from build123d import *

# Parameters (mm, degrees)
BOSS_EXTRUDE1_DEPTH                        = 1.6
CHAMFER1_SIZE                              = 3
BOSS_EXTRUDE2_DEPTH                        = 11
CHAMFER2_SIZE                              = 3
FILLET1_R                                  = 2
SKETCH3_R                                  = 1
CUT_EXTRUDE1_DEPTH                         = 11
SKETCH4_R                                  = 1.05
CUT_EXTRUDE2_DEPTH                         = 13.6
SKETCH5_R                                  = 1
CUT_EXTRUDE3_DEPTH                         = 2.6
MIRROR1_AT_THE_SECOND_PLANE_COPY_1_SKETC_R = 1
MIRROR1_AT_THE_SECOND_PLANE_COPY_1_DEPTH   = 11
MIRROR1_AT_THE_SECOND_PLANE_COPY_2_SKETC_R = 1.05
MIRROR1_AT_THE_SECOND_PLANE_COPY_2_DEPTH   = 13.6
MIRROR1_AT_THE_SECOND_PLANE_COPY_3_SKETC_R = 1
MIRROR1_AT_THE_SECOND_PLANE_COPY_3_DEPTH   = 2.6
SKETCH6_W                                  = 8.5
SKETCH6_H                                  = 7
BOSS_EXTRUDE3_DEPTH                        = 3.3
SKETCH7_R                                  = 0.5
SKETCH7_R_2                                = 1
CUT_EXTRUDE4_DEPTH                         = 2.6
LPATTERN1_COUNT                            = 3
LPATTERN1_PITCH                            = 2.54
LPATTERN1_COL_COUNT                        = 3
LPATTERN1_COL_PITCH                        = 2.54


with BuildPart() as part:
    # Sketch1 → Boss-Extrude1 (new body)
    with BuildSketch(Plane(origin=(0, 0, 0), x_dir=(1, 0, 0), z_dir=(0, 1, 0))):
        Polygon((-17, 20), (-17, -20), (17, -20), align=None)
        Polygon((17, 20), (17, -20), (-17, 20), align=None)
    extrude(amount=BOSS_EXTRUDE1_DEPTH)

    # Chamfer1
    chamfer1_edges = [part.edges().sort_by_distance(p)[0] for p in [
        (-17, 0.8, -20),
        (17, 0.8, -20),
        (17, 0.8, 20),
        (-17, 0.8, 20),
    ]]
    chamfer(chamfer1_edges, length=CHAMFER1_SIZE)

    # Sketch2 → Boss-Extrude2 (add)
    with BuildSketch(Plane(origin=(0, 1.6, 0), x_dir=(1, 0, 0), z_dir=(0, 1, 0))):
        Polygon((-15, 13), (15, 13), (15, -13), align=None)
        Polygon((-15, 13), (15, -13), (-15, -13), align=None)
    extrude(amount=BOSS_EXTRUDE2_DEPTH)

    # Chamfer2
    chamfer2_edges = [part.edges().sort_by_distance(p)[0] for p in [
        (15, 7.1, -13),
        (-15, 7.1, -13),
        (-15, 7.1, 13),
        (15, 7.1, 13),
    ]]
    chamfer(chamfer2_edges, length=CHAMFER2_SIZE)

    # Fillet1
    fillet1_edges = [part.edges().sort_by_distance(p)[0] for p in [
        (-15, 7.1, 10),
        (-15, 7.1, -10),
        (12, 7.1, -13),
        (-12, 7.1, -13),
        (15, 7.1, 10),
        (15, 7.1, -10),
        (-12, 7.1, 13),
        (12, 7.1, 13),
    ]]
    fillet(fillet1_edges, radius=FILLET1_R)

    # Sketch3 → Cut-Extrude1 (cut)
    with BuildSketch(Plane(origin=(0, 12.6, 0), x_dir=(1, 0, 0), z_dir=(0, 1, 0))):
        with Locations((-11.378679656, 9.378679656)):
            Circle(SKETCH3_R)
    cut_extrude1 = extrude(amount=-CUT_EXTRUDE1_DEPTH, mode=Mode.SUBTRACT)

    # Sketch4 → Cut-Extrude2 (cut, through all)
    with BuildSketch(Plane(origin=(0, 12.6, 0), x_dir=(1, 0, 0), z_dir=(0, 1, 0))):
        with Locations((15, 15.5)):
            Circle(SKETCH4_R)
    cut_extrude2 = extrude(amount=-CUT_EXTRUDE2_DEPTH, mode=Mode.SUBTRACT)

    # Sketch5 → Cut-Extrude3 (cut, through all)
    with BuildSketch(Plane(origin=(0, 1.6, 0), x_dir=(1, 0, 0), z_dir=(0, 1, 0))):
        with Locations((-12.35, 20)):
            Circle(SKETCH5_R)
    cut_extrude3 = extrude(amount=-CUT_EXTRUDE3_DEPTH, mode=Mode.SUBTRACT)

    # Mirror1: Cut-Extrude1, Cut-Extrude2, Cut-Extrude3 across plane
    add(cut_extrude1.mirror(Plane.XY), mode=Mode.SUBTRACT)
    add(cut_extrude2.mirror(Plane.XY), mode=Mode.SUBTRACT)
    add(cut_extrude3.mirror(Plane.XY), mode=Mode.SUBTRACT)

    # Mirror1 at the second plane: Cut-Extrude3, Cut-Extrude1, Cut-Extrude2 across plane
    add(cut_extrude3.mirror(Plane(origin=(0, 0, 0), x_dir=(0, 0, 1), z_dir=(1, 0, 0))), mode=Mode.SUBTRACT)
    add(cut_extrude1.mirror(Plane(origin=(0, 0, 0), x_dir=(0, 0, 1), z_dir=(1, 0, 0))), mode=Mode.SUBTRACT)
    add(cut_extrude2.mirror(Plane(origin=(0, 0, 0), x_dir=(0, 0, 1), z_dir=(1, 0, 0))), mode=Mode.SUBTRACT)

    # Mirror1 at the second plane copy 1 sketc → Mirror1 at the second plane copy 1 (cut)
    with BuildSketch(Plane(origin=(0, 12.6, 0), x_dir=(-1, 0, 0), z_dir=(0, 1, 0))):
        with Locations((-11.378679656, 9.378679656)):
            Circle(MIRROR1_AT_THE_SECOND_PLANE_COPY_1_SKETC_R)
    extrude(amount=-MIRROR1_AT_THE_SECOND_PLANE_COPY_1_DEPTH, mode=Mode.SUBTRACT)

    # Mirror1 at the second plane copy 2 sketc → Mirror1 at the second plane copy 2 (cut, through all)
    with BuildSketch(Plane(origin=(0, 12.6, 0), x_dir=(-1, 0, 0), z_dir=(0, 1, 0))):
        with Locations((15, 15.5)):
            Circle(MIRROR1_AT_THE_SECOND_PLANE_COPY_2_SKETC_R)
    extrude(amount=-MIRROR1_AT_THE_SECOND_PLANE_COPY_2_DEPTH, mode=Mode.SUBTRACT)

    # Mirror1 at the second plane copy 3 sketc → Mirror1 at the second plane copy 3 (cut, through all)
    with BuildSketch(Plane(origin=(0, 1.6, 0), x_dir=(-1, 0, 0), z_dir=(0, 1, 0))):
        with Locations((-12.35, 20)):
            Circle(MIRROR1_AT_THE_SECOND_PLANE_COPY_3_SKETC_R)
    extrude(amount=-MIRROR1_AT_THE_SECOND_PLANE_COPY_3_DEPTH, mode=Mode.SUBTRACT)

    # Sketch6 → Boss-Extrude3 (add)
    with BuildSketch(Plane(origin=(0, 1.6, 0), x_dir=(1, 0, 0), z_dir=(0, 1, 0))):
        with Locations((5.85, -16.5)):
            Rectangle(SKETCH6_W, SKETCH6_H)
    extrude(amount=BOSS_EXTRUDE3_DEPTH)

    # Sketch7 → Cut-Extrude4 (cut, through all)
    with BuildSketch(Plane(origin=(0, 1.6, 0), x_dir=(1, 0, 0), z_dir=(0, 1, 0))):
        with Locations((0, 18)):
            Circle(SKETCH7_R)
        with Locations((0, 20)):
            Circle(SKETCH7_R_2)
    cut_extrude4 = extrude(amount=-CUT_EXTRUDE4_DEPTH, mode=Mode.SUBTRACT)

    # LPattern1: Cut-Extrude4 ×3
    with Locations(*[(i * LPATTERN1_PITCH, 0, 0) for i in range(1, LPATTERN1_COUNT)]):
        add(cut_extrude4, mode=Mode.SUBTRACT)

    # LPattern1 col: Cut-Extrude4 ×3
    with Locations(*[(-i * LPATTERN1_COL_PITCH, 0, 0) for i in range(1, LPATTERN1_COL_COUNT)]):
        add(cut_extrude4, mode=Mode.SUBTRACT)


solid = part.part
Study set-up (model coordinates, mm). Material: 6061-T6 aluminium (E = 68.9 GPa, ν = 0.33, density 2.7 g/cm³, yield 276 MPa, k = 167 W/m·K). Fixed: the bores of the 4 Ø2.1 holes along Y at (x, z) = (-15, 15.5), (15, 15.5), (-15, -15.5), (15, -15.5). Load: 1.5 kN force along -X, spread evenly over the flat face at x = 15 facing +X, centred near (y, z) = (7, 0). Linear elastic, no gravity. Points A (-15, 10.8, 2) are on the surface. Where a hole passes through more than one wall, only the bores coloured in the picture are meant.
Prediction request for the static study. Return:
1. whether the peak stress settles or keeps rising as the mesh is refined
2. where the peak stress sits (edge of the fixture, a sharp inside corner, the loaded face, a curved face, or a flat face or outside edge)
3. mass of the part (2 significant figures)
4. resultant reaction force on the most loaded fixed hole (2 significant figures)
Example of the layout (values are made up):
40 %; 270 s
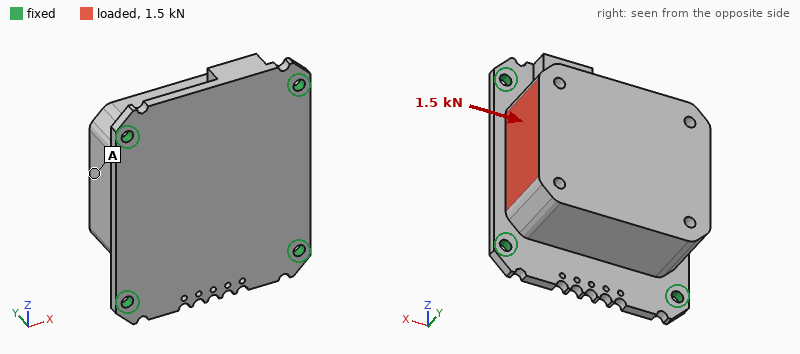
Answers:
keeps rising; edge of the fixture; 28 g; 480 N
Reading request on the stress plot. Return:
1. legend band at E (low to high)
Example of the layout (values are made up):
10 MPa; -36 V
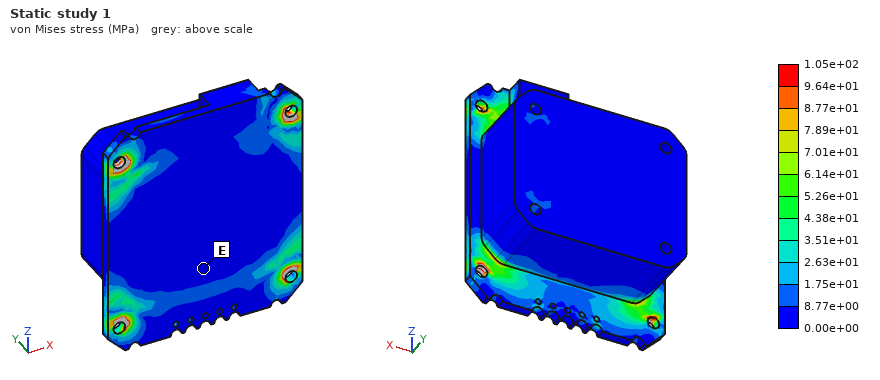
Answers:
0.00e+00 to 8.77e+00 MPa
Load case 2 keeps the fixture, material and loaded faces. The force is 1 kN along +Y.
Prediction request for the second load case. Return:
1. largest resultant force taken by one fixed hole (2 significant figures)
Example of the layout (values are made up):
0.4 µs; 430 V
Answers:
580 N
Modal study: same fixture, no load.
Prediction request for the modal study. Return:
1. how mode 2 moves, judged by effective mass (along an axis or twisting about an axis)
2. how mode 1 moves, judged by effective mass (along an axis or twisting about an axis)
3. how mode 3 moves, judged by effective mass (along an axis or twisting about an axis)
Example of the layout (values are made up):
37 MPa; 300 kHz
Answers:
along X; along Y; along Z
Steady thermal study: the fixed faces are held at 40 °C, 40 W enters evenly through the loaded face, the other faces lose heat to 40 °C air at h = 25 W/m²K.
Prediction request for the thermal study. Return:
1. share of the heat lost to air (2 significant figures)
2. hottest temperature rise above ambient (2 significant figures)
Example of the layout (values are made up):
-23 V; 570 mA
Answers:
5.3 %; 34 K
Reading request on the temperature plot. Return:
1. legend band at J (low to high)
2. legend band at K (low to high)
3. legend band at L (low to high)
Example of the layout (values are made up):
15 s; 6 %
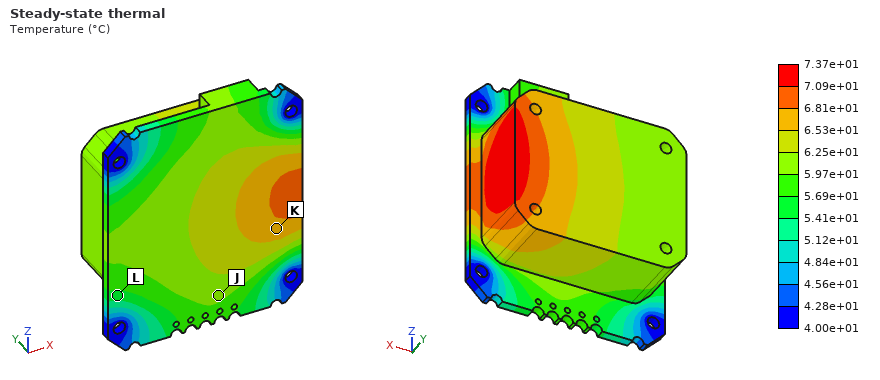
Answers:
5.97e+01 to 6.25e+01 °C; 6.53e+01 to 6.81e+01 °C; 5.41e+01 to 5.69e+01 °C
